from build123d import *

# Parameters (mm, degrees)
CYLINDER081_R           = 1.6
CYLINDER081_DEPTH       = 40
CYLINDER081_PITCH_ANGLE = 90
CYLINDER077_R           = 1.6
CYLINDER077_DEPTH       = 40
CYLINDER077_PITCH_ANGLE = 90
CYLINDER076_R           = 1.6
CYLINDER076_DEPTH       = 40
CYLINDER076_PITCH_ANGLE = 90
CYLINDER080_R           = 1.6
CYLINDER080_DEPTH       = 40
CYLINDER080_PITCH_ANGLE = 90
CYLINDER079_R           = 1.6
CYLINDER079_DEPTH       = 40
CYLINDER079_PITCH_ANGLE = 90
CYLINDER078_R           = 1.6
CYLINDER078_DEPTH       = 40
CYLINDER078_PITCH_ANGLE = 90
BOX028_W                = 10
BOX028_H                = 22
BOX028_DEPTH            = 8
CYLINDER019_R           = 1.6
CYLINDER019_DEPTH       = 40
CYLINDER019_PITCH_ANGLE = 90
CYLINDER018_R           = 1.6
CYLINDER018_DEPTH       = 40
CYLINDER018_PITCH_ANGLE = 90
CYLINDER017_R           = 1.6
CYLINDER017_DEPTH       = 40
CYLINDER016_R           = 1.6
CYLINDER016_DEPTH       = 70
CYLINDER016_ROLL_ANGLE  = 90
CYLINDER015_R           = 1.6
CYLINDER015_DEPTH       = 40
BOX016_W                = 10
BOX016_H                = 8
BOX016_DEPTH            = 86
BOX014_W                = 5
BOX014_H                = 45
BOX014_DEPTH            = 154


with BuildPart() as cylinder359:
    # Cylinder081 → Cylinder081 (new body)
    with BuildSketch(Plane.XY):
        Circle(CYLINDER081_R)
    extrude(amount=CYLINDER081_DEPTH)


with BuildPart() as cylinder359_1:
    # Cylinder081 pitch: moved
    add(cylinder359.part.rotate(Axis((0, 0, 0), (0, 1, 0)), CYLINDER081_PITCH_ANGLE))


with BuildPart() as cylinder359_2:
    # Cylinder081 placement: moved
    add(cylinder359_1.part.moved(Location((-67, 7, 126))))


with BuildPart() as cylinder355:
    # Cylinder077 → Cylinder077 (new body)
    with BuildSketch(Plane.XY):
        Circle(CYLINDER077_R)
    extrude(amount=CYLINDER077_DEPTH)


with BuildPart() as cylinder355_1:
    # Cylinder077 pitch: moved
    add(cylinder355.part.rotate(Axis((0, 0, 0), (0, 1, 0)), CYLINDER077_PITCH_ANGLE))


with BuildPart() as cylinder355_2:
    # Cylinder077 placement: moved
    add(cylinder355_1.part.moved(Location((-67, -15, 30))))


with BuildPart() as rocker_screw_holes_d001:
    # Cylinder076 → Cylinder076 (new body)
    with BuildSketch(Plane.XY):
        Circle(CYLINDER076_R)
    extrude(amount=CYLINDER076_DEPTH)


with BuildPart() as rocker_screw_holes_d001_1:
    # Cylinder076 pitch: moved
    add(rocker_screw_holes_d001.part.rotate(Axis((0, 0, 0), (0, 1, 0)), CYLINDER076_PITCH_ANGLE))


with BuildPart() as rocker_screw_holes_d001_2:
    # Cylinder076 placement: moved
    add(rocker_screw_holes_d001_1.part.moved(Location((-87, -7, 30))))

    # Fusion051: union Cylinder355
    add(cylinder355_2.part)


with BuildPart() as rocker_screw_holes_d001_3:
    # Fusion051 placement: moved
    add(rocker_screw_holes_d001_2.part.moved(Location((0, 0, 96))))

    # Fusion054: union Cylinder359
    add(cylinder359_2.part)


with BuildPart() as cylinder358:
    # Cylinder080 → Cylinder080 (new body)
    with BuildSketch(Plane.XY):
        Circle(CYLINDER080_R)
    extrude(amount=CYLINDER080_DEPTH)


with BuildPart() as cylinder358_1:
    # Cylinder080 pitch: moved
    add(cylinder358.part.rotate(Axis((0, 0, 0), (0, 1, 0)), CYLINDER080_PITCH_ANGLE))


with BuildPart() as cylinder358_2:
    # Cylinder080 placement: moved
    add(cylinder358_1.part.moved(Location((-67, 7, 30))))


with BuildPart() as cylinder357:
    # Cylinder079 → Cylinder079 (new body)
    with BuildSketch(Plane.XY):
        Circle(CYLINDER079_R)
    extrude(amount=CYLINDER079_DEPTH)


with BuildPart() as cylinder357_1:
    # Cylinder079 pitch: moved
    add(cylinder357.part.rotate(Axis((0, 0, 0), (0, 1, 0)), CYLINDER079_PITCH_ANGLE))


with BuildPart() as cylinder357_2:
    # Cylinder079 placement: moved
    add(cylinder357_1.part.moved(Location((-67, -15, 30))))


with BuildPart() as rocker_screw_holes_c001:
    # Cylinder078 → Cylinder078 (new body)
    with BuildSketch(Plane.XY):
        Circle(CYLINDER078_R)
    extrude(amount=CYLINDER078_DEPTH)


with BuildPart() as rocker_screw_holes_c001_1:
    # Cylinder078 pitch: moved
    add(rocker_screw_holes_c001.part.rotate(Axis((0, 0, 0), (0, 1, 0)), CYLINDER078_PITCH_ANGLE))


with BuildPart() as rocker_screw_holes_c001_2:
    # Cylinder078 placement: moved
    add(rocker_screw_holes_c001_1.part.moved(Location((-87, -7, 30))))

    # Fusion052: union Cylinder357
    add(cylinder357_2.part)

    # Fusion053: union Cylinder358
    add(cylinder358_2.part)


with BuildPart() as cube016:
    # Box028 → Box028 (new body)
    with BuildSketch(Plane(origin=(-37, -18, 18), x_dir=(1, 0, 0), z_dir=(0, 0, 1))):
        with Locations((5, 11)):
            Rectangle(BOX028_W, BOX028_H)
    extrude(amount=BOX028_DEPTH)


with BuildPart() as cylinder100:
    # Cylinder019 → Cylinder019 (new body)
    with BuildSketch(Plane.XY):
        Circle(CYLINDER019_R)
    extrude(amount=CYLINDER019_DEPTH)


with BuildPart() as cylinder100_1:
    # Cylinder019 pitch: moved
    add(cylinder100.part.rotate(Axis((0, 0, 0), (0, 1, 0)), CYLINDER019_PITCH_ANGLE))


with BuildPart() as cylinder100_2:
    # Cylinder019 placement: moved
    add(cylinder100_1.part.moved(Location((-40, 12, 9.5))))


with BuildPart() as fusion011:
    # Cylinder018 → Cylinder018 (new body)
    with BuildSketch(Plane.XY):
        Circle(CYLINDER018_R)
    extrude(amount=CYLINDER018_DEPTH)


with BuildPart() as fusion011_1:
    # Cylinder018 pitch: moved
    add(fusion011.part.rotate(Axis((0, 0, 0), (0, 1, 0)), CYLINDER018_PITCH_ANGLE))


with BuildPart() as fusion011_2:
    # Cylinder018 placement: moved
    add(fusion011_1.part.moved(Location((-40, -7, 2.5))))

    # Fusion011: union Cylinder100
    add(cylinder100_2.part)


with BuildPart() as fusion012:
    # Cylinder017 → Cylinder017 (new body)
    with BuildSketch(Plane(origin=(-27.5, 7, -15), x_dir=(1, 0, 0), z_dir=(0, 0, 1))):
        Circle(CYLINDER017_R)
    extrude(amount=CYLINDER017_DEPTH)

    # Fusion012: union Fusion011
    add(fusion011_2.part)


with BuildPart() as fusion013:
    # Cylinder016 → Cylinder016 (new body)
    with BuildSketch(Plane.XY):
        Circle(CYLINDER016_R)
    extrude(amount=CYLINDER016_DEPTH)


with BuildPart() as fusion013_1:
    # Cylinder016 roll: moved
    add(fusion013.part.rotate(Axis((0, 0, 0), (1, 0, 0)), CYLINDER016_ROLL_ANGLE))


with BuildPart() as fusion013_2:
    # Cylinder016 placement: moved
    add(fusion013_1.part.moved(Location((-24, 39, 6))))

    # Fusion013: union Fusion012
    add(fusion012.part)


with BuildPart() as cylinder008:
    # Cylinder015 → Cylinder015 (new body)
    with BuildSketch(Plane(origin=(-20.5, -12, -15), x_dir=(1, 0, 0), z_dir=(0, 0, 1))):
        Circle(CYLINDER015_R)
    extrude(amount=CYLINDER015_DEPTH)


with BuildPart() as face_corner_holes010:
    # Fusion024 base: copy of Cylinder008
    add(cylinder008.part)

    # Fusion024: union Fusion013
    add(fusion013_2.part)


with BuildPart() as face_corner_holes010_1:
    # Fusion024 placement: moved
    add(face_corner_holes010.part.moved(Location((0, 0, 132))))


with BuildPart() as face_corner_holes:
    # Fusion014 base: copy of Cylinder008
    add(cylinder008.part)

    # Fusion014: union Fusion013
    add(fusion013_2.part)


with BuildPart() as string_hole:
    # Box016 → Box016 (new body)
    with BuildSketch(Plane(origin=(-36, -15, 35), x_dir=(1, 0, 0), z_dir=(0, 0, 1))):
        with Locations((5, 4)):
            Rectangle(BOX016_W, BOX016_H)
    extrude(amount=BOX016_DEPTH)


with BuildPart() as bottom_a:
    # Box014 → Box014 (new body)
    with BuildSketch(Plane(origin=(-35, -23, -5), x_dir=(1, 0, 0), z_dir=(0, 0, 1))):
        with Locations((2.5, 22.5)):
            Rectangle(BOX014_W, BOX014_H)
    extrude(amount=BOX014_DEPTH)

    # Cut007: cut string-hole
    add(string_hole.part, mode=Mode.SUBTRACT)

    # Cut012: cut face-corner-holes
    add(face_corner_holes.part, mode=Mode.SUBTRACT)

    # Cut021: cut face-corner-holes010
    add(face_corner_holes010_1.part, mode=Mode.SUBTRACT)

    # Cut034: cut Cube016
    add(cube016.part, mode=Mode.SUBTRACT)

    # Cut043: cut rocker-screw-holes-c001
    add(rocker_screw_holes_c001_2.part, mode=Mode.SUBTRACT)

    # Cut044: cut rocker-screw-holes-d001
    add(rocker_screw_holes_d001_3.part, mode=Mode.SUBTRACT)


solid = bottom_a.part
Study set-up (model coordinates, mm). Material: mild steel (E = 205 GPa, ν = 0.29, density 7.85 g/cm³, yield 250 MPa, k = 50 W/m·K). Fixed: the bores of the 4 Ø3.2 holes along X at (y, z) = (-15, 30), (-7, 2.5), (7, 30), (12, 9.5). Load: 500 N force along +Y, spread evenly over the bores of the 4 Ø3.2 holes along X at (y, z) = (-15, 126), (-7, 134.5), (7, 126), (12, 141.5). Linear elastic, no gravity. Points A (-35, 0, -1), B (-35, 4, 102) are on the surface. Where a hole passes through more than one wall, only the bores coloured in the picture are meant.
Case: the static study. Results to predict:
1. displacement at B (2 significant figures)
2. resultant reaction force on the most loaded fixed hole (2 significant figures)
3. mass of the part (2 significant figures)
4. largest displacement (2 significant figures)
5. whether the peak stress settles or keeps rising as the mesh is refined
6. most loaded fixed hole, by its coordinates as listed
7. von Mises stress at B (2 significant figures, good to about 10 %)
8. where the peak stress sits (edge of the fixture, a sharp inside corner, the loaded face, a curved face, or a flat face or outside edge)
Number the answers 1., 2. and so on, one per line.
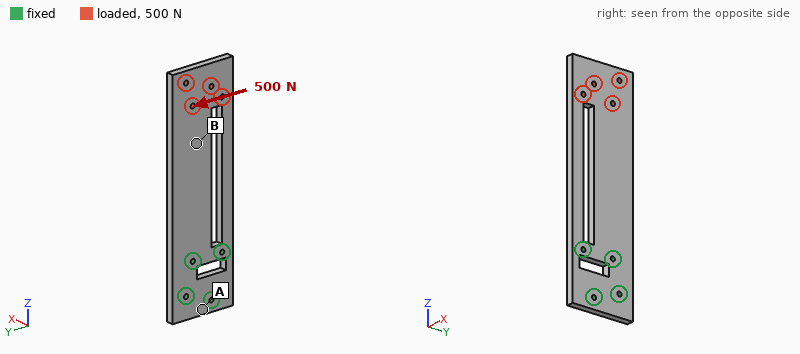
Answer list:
1. 40 µm
2. 1.4 kN
3. 240 g
4. 68 µm
5. keeps rising
6. (-15, 30)
7. 10 MPa
8. edge of the fixture
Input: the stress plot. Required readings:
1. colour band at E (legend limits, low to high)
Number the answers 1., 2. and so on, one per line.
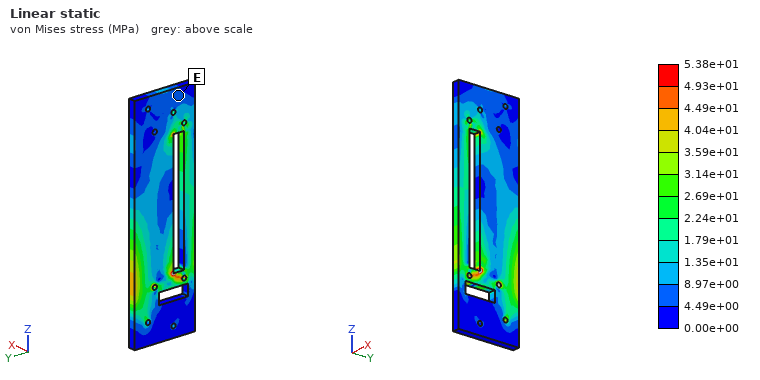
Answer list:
1. 4.49e+00 to 8.97e+00 MPa
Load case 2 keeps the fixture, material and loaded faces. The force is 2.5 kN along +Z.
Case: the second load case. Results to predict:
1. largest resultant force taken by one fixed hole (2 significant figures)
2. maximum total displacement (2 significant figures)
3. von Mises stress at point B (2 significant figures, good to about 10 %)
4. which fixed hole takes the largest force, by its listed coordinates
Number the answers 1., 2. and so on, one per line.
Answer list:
1. 1.3 kN
2. 12 µm
3. 13 MPa
4. (7, 30)
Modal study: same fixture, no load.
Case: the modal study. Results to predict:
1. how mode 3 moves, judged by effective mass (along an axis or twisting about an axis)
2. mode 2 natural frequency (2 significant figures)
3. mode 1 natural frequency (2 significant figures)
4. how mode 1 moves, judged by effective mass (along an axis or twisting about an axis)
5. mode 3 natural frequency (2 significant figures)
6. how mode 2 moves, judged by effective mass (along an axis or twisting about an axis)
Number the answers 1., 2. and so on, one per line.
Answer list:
1. along Y
2. 1300 Hz
3. 270 Hz
4. along X
5. 1600 Hz
6. twisting about Z
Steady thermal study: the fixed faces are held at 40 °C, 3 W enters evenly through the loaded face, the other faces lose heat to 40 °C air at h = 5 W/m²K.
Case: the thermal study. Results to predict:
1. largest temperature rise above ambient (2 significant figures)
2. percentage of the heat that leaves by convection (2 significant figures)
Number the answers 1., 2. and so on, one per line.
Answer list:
1. 27 K
2. 29 %
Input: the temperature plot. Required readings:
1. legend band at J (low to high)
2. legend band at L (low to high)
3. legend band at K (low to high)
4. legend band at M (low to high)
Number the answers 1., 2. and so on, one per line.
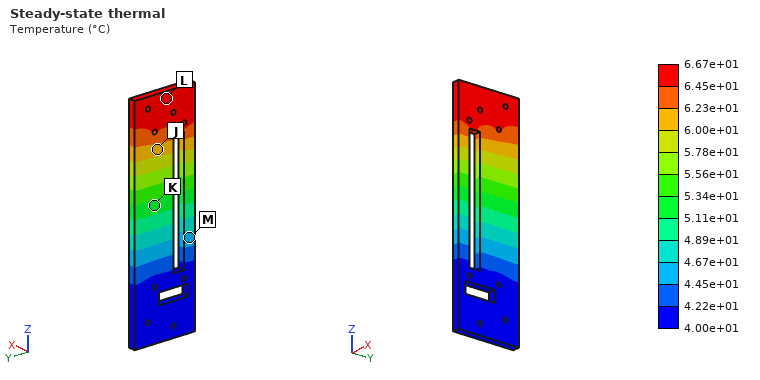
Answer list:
1. 6.00e+01 to 6.23e+01 °C
2. 6.45e+01 to 6.67e+01 °C
3. 5.11e+01 to 5.34e+01 °C
4. 4.45e+01 to 4.67e+01 °C
